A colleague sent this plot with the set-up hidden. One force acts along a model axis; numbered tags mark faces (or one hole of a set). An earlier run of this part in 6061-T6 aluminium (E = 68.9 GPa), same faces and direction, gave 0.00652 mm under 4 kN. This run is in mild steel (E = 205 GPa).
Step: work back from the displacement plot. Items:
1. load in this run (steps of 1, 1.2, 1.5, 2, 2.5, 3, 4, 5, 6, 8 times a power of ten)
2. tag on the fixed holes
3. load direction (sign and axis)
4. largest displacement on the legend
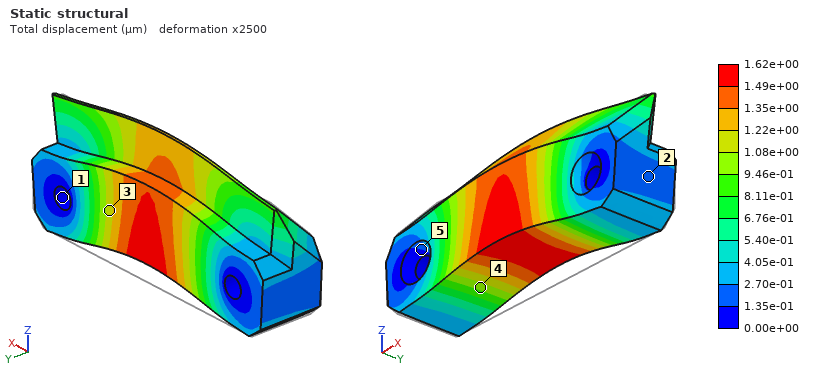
3 kN
1
+Z
1.62e+00 µm
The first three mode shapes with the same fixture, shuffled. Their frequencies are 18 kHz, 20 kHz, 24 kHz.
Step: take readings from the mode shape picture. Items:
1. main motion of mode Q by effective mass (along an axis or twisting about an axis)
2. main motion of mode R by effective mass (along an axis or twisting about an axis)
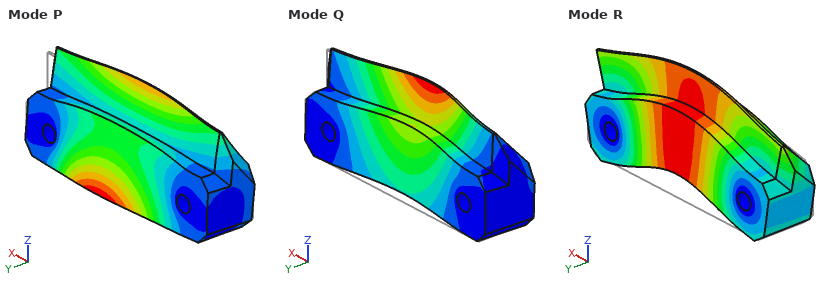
along Y
along Z
